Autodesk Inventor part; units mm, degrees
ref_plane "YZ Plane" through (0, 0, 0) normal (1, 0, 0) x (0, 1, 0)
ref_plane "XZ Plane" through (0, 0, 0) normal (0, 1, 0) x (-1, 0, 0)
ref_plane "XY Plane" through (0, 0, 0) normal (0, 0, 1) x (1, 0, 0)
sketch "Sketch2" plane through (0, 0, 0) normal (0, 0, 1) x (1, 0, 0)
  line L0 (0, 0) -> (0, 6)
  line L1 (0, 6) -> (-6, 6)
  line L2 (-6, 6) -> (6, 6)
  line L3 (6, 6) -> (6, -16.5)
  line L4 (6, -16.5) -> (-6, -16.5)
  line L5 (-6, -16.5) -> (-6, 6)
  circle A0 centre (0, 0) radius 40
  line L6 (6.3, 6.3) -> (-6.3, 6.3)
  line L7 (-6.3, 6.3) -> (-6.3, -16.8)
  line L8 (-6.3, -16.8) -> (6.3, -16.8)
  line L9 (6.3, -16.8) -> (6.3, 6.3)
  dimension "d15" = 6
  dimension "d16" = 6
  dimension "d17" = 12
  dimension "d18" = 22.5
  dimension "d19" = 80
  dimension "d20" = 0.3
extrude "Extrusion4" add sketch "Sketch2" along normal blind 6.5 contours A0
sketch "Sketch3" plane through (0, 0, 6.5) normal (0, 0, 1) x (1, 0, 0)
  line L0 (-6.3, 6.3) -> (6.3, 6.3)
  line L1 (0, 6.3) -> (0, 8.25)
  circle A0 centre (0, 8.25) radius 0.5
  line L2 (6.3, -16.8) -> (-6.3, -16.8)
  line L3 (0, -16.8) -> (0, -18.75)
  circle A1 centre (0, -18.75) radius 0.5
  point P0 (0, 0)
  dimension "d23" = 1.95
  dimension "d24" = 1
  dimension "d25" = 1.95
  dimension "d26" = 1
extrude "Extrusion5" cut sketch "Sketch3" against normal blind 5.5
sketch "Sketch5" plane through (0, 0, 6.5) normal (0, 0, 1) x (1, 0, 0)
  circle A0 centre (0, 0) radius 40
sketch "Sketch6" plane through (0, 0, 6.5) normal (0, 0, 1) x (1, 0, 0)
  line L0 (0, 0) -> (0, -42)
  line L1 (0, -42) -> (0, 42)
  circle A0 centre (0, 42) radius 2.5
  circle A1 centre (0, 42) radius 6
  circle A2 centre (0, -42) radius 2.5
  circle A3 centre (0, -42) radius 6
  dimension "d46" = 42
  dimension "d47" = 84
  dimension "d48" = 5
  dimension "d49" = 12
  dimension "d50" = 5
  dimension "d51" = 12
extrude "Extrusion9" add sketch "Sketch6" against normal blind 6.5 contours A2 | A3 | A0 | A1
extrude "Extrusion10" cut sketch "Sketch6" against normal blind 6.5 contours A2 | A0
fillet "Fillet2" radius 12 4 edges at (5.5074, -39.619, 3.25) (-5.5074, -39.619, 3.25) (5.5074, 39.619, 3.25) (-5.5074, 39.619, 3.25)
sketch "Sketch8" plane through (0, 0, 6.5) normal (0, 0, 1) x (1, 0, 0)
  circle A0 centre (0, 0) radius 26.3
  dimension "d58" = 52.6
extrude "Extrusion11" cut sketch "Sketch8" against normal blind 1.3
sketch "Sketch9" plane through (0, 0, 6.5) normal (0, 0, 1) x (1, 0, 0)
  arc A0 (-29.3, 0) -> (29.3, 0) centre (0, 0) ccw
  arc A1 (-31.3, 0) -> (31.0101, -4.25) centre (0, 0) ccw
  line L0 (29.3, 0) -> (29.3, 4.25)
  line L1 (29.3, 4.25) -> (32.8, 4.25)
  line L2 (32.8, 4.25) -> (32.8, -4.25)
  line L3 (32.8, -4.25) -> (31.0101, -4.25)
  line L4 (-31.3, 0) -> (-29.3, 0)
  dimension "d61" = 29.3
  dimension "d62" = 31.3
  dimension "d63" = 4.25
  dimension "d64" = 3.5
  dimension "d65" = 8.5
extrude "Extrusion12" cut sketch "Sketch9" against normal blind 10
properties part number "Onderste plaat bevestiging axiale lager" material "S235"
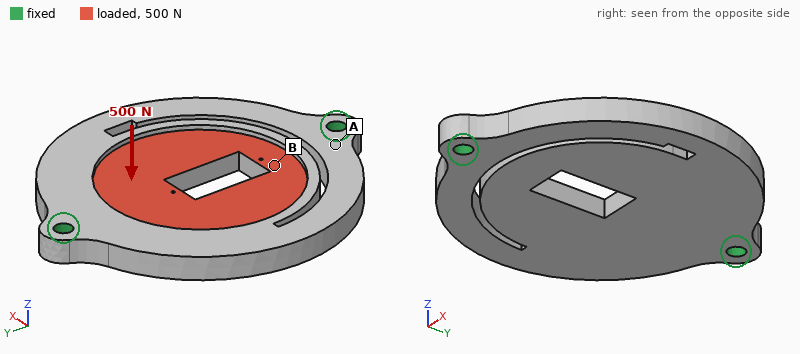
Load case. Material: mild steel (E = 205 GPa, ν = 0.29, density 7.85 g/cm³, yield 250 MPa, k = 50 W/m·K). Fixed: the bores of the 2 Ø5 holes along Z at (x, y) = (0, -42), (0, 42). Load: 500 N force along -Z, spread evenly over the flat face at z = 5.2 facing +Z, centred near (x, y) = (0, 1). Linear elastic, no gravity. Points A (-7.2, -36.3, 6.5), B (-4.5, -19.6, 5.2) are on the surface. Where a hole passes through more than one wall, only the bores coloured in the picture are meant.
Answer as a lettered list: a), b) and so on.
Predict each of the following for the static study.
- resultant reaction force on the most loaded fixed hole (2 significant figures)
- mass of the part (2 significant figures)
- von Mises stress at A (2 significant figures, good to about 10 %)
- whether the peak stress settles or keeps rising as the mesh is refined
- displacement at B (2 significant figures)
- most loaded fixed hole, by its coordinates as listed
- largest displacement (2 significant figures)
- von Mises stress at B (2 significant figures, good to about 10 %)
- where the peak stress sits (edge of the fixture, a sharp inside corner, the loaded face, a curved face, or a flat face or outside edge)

a) 310 N
b) 220 g
c) 27 MPa
d) keeps rising
e) 63 µm
f) (0, 42)
g) 77 µm
h) 9.1 MPa
i) edge of the fixture
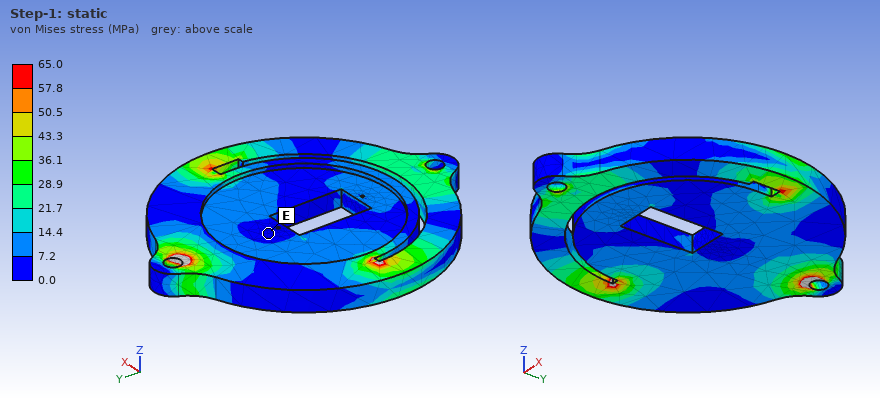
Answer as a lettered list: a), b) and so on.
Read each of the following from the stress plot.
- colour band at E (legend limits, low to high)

a) 0.0 to 7.2 MPa
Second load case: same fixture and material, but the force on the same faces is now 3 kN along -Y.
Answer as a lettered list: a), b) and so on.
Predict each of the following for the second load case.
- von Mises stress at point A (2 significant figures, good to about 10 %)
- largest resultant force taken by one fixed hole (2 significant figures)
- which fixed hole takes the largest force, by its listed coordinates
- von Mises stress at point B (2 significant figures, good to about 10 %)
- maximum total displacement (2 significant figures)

a) 6.3 MPa
b) 2.7 kN
c) (0, 42)
d) 9.1 MPa
e) 45 µm
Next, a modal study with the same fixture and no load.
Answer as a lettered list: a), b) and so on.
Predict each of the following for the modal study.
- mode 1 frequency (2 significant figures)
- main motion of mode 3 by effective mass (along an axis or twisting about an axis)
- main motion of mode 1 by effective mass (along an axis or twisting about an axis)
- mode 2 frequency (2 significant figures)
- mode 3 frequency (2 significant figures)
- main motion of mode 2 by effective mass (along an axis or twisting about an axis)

a) 1500 Hz
b) along Z
c) along Z
d) 1800 Hz
e) 3400 Hz
f) twisting about Y
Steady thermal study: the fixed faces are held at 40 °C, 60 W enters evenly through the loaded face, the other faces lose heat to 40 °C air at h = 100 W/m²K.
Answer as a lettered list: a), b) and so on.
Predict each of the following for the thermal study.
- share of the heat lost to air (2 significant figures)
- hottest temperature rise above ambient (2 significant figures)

a) 69 %
b) 77 K
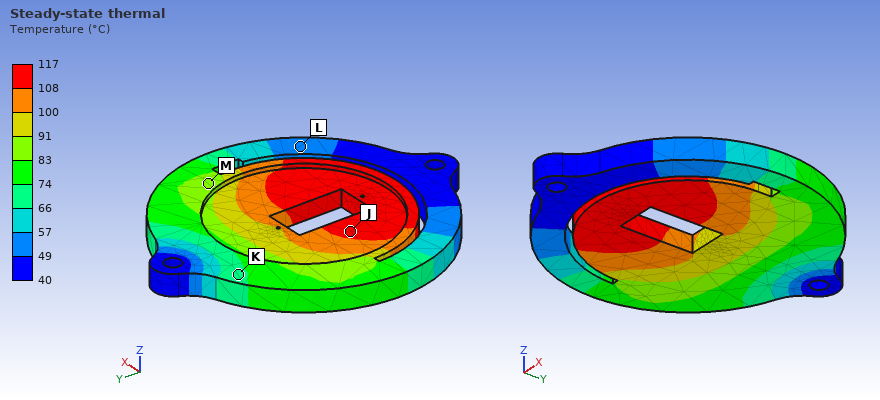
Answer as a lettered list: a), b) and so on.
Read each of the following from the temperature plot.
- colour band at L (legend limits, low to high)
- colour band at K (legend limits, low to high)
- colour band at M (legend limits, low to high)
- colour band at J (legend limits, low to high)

a) 49 to 57 °C
b) 66 to 74 °C
c) 83 to 91 °C
d) 108 to 117 °C
